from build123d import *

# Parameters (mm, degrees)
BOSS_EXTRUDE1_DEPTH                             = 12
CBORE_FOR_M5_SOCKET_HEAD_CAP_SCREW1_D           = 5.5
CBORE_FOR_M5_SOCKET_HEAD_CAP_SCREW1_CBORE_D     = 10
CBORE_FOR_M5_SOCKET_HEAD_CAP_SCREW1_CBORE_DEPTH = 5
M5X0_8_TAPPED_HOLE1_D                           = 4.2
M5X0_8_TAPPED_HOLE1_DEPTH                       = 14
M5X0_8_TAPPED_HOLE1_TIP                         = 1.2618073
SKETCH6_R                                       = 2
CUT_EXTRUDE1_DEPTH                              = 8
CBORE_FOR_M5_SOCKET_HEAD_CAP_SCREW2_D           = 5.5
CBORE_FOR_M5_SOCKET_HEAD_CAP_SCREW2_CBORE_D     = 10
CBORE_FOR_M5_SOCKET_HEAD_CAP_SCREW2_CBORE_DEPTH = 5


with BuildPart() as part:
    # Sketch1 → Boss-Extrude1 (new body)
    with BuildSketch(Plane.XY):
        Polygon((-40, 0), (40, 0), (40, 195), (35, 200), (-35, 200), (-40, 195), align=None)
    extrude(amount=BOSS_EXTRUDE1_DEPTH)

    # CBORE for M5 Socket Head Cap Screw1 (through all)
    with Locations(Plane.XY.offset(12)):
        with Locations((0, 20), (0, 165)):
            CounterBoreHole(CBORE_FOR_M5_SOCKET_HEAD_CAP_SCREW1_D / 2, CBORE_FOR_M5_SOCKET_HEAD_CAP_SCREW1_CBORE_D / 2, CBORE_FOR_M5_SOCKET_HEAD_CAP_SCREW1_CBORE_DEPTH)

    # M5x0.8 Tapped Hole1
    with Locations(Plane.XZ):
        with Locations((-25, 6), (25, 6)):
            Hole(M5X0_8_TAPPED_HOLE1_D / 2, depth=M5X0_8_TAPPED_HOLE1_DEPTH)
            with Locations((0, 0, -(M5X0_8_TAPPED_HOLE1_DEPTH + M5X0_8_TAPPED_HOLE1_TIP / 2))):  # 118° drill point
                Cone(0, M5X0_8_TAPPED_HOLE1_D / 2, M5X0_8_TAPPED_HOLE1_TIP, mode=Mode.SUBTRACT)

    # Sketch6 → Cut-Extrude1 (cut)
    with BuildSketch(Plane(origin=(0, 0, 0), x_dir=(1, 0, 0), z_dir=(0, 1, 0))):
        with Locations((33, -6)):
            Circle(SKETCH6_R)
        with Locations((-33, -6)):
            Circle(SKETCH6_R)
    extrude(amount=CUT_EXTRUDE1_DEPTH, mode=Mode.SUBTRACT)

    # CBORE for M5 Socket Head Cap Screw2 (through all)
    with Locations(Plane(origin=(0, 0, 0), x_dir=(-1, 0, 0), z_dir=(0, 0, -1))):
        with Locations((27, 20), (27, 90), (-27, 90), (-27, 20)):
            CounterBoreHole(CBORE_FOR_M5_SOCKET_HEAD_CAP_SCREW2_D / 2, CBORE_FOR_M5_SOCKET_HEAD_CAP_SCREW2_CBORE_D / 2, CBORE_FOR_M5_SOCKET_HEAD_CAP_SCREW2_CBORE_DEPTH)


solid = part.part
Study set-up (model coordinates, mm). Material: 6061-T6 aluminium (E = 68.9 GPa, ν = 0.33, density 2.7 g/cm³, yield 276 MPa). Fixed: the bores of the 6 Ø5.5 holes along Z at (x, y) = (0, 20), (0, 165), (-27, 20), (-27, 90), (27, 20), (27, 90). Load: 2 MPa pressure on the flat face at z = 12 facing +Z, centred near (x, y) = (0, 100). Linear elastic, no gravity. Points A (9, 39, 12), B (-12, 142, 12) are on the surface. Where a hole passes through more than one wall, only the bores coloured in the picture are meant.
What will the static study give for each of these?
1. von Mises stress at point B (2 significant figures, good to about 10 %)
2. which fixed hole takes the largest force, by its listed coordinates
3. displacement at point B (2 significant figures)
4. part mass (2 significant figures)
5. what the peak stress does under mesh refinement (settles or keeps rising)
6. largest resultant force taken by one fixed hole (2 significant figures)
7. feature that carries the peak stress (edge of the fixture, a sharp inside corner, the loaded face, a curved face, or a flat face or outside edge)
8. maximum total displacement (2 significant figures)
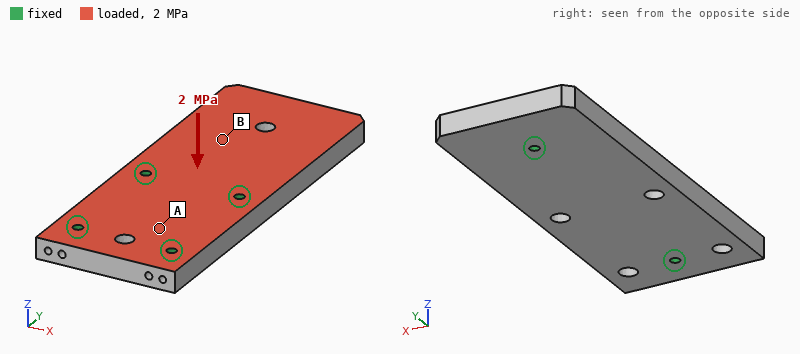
29 MPa
(0, 165)
0.036 mm
510 g
keeps rising
12 kN
edge of the fixture
0.12 mm
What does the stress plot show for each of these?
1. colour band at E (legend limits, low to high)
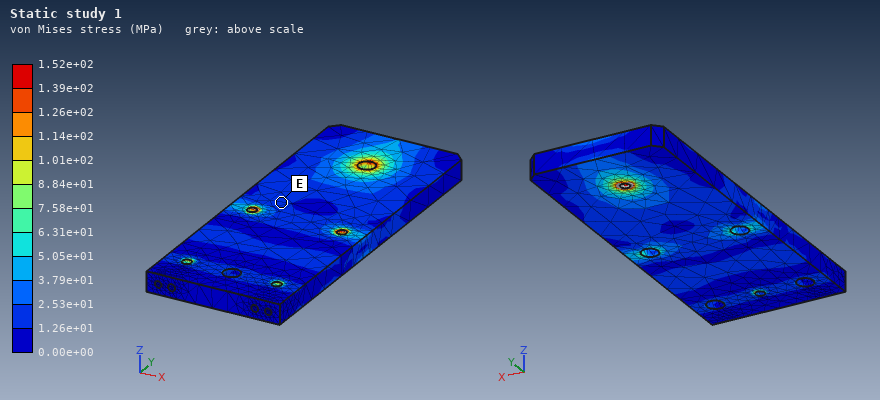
1.26e+01 to 2.53e+01 MPa
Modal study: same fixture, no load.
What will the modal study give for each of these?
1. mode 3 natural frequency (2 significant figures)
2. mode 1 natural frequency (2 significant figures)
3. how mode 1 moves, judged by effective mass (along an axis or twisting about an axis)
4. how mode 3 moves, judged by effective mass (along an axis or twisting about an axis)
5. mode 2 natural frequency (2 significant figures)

5500 Hz
3000 Hz
twisting about Y
along Z
4200 Hz
